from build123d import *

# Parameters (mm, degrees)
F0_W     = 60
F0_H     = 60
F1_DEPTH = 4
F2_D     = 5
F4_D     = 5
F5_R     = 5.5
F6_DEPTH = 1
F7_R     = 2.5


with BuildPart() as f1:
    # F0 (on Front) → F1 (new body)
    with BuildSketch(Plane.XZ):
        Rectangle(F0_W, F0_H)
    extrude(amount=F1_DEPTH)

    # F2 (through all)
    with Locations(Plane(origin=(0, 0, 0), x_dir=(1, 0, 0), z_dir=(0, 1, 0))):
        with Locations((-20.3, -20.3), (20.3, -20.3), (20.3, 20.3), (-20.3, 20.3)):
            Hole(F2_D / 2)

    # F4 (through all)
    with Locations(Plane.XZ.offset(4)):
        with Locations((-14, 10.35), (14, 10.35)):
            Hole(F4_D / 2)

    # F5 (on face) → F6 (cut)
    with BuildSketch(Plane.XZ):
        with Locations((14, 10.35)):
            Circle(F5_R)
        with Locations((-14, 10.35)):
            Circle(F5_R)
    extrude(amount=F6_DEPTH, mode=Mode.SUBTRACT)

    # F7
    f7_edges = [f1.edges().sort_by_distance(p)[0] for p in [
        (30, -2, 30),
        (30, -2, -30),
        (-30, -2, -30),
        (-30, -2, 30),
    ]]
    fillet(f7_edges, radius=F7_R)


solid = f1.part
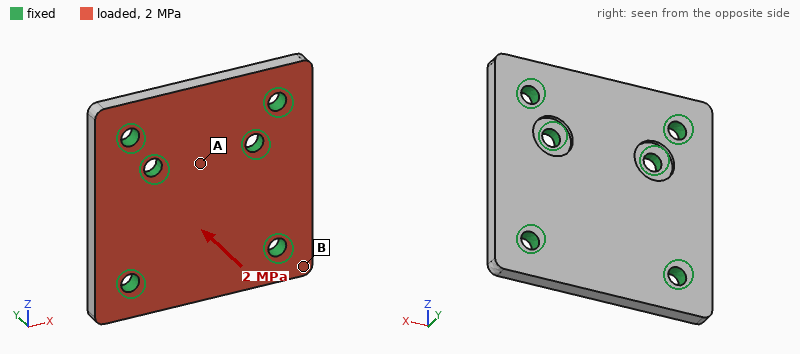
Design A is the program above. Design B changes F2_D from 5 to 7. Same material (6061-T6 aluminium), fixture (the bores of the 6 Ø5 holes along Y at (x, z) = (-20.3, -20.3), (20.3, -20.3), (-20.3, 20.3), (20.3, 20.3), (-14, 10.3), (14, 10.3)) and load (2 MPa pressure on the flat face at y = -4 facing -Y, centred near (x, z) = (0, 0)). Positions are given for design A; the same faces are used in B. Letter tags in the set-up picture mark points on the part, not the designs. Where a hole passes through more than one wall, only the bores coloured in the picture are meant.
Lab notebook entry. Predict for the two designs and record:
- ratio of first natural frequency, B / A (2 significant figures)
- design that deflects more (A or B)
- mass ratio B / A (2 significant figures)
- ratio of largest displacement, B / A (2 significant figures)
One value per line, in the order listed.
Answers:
1.1
A
0.98
0.77
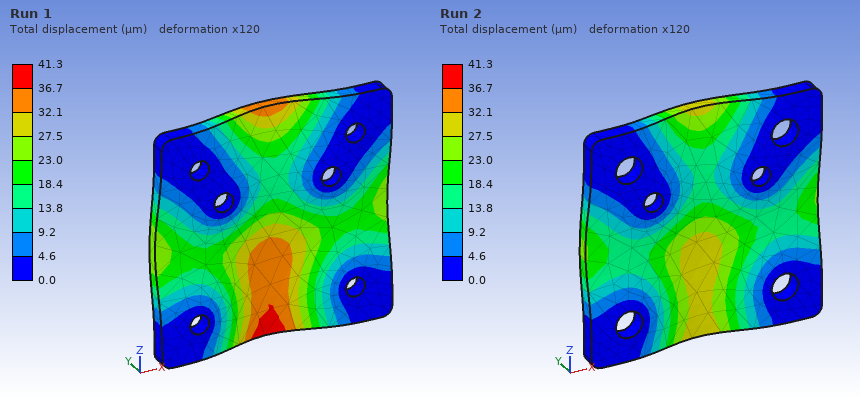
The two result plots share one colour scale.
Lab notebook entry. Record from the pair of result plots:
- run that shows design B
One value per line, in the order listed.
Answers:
Run 2
